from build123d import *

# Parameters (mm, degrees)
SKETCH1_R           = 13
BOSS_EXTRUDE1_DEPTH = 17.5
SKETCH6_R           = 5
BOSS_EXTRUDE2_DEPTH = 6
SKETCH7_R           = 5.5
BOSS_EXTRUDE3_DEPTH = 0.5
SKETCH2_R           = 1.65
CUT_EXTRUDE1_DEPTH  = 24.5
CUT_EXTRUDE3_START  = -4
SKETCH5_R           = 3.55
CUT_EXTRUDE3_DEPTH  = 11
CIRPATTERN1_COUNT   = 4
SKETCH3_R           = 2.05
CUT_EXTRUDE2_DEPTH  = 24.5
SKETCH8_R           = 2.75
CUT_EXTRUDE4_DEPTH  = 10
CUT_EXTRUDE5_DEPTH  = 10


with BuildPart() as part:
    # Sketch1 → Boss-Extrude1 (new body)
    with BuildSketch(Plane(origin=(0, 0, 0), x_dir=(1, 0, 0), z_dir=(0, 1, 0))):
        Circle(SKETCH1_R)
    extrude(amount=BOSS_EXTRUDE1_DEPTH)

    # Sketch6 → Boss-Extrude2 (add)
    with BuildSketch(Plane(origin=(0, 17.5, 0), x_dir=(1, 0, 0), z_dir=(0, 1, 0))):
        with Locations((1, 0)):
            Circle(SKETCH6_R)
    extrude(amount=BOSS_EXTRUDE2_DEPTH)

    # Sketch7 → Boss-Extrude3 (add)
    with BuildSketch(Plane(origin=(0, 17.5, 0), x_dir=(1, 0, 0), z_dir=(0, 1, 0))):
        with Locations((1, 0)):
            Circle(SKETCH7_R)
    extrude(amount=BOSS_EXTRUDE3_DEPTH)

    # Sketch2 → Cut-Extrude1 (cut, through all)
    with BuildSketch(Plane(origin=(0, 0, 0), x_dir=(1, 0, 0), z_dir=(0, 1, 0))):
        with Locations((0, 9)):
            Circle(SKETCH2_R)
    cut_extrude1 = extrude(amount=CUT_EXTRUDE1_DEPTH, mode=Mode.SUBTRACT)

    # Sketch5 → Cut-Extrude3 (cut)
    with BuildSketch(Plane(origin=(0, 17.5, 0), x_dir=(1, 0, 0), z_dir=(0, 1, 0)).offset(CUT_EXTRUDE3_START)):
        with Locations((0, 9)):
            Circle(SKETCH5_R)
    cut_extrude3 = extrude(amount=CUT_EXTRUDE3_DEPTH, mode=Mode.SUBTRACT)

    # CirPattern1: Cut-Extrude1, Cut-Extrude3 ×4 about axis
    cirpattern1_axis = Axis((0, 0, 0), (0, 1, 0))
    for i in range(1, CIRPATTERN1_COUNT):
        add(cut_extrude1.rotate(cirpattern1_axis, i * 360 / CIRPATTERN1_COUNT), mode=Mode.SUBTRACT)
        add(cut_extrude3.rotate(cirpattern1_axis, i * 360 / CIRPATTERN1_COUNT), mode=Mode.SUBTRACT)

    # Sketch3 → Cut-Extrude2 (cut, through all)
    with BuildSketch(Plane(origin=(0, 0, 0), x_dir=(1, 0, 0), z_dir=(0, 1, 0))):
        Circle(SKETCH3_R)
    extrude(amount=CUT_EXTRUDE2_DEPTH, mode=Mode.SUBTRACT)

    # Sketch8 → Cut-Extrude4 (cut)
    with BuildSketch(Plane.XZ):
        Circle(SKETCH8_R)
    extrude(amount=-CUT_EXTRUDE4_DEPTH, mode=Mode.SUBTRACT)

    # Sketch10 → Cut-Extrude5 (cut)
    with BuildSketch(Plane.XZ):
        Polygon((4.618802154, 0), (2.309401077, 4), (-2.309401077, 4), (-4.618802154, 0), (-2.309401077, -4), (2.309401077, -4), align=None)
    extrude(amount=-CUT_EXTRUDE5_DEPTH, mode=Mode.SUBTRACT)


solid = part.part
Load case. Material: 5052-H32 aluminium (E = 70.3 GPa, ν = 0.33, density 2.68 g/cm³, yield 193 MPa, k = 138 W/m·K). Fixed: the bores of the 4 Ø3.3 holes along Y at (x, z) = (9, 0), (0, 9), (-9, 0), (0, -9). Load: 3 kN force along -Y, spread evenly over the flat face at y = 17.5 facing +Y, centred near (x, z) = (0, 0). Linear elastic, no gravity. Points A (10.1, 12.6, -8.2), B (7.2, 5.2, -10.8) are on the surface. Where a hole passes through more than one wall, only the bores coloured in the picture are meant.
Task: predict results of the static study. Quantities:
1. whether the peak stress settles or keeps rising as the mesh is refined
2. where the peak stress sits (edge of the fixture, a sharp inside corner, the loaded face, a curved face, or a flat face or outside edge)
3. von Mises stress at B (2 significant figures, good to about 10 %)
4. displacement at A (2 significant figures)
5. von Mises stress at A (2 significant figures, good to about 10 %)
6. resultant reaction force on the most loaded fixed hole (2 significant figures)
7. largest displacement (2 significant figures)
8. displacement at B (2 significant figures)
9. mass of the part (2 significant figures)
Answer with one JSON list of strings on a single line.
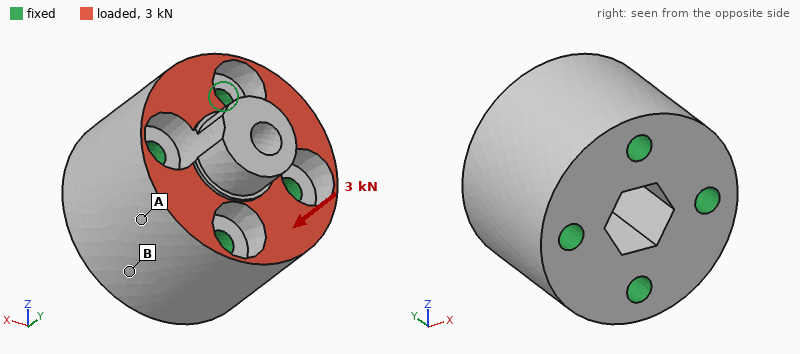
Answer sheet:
["keeps rising", "edge of the fixture", "3.0 MPa", "1.2 µm", "8.4 MPa", "800 N", "2.1 µm", "0.51 µm", "21 g"]
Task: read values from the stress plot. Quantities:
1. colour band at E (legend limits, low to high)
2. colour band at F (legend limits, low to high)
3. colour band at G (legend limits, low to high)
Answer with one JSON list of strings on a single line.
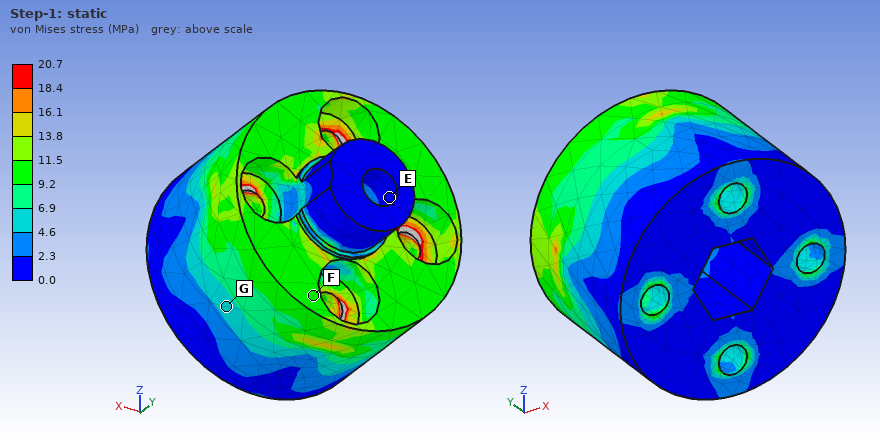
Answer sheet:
["0.0 to 2.3 MPa", "9.2 to 11.5 MPa", "4.6 to 6.9 MPa"]
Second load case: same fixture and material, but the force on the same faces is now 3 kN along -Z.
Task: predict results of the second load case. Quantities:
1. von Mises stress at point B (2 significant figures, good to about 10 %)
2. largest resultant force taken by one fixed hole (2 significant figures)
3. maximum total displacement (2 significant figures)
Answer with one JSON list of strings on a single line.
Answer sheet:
["4.9 MPa", "1.1 kN", "8.3 µm"]
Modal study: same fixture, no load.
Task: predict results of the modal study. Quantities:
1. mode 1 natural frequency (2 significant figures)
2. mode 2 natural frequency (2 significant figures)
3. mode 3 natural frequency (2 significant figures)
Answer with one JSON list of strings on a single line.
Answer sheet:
["56 kHz", "57 kHz", "83 kHz"]
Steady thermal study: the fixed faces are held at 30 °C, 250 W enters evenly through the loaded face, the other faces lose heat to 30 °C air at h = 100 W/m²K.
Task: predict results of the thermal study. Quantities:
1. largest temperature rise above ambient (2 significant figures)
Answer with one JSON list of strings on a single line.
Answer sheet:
["47 K"]
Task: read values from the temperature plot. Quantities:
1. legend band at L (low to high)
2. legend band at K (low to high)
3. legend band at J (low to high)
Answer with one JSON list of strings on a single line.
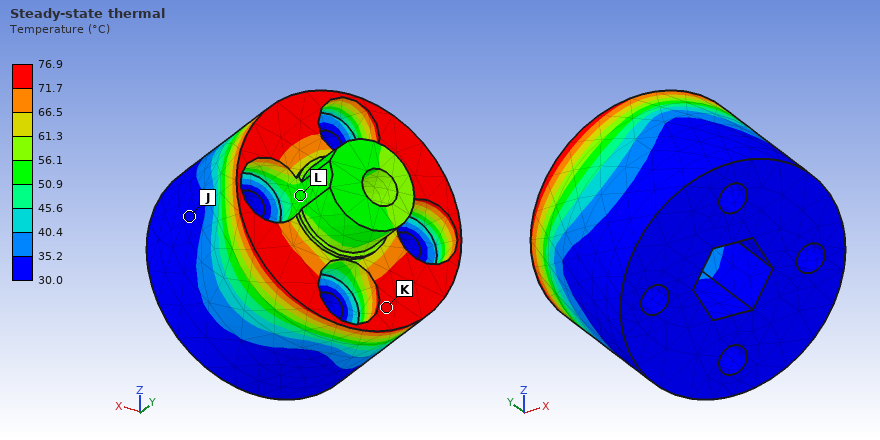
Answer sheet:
["50.9 to 56.1 °C", "71.7 to 76.9 °C", "30.0 to 35.2 °C"]
